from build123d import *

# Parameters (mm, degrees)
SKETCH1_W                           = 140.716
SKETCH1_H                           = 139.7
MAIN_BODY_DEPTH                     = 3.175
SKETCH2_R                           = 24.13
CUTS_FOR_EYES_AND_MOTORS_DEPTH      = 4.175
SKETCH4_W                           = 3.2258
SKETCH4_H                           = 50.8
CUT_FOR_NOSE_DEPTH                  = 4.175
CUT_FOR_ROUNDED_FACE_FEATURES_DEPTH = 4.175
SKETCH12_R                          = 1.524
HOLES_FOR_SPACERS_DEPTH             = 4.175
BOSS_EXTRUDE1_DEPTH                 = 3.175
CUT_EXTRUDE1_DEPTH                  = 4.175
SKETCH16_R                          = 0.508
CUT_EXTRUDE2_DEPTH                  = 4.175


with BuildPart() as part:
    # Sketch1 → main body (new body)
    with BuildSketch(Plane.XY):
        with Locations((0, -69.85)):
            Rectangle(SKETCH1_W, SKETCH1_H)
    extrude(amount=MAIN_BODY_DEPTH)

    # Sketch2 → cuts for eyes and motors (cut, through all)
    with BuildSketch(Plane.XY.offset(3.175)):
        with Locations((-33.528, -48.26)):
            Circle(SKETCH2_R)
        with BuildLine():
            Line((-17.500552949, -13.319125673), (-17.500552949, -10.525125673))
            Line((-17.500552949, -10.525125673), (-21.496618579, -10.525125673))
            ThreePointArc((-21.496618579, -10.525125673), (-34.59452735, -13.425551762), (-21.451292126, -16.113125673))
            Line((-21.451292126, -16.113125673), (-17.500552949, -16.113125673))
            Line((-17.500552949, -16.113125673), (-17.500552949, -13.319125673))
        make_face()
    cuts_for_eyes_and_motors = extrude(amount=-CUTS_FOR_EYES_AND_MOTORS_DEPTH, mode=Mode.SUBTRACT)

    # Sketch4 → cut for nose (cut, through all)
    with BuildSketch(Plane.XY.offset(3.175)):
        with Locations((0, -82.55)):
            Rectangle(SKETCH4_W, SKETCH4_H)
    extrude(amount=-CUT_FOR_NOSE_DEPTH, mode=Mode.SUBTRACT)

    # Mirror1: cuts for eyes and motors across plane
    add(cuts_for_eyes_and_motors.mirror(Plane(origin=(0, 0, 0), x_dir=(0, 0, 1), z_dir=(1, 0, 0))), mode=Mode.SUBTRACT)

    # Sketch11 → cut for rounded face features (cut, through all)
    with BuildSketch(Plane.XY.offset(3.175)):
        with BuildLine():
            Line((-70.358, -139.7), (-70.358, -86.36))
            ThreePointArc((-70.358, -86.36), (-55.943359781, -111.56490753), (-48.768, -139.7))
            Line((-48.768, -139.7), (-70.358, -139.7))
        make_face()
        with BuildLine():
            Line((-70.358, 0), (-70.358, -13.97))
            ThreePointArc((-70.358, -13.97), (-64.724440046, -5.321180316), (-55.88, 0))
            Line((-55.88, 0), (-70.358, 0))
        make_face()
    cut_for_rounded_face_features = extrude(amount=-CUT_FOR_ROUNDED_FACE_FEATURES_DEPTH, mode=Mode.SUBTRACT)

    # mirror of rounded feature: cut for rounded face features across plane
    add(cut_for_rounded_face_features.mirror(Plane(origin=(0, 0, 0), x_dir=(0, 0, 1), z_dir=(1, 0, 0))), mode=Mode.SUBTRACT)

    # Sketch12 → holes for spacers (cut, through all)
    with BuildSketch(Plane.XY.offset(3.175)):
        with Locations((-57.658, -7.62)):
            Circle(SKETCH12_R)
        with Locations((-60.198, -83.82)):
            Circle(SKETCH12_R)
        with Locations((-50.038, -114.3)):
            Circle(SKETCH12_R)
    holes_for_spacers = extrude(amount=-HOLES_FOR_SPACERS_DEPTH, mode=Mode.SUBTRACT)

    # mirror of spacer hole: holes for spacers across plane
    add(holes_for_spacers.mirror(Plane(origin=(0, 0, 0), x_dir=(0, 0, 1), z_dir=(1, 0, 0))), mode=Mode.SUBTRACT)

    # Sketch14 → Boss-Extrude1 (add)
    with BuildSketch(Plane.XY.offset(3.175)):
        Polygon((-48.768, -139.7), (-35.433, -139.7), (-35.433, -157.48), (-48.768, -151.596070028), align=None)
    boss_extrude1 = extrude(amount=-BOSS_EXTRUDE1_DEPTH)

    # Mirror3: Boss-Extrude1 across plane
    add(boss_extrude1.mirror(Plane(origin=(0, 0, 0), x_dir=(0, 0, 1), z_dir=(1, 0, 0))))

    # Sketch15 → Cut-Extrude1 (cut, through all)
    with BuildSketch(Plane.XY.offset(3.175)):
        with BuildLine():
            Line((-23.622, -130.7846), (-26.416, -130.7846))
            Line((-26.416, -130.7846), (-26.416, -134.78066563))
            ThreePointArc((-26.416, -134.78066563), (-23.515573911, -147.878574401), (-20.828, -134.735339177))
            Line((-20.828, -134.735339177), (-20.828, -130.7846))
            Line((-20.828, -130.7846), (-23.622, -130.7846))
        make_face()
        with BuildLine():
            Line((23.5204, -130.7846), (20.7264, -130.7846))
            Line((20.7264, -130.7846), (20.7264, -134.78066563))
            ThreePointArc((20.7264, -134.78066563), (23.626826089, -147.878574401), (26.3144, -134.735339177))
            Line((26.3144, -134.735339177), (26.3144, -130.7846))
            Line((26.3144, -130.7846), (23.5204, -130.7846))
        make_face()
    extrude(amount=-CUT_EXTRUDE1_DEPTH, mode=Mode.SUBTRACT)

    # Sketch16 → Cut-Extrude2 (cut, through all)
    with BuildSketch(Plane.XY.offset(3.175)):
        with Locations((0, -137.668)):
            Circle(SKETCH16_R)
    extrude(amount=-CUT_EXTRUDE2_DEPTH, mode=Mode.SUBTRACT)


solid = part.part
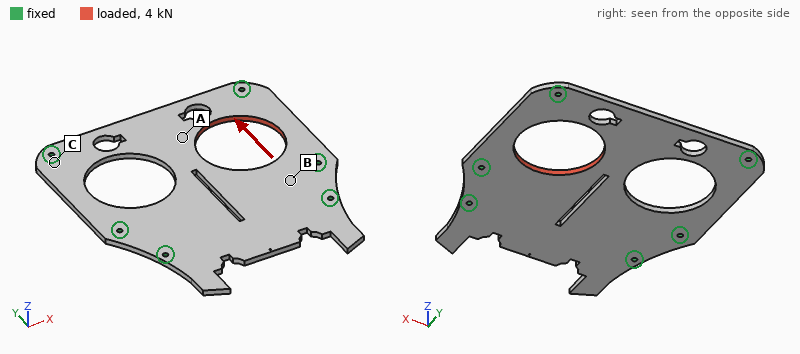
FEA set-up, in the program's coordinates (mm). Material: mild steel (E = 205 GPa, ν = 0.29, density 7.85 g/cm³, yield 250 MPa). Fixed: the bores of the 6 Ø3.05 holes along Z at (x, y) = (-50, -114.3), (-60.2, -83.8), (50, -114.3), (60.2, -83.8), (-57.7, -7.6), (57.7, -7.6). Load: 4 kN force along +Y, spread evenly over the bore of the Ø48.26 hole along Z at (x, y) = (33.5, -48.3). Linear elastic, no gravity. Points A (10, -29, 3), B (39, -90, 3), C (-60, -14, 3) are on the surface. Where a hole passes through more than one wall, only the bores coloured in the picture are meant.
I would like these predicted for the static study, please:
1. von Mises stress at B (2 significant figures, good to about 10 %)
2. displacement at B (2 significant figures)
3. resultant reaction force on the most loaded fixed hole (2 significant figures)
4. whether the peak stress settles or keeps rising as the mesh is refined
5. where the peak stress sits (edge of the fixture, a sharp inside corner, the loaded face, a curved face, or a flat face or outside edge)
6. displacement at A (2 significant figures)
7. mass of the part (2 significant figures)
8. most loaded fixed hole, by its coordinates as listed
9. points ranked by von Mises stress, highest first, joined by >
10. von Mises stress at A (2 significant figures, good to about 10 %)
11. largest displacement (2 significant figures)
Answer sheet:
13 MPa
2.4 µm
1.2 kN
keeps rising
edge of the fixture
7.5 µm
350 g
(57.7, -7.6)
B > A > C
5.8 MPa
9.1 µm
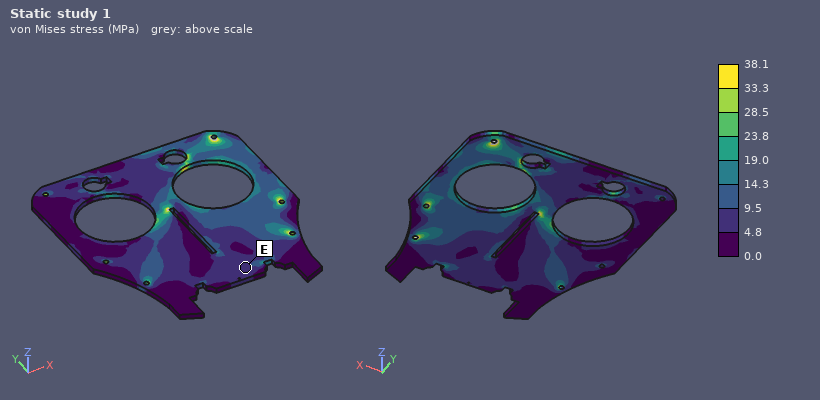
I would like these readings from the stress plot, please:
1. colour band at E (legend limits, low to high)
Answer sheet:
4.8 to 9.5 MPa
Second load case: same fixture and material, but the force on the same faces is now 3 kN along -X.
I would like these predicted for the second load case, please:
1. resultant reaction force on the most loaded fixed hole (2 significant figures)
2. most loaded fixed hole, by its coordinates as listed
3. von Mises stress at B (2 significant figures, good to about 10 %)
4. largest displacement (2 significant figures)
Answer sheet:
1.2 kN
(60.2, -83.8)
10 MPa
8.5 µm
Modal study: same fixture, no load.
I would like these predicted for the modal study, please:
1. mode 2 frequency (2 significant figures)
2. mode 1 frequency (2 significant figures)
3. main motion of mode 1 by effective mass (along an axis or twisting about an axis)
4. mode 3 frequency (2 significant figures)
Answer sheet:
1300 Hz
1000 Hz
along Z
1600 Hz
